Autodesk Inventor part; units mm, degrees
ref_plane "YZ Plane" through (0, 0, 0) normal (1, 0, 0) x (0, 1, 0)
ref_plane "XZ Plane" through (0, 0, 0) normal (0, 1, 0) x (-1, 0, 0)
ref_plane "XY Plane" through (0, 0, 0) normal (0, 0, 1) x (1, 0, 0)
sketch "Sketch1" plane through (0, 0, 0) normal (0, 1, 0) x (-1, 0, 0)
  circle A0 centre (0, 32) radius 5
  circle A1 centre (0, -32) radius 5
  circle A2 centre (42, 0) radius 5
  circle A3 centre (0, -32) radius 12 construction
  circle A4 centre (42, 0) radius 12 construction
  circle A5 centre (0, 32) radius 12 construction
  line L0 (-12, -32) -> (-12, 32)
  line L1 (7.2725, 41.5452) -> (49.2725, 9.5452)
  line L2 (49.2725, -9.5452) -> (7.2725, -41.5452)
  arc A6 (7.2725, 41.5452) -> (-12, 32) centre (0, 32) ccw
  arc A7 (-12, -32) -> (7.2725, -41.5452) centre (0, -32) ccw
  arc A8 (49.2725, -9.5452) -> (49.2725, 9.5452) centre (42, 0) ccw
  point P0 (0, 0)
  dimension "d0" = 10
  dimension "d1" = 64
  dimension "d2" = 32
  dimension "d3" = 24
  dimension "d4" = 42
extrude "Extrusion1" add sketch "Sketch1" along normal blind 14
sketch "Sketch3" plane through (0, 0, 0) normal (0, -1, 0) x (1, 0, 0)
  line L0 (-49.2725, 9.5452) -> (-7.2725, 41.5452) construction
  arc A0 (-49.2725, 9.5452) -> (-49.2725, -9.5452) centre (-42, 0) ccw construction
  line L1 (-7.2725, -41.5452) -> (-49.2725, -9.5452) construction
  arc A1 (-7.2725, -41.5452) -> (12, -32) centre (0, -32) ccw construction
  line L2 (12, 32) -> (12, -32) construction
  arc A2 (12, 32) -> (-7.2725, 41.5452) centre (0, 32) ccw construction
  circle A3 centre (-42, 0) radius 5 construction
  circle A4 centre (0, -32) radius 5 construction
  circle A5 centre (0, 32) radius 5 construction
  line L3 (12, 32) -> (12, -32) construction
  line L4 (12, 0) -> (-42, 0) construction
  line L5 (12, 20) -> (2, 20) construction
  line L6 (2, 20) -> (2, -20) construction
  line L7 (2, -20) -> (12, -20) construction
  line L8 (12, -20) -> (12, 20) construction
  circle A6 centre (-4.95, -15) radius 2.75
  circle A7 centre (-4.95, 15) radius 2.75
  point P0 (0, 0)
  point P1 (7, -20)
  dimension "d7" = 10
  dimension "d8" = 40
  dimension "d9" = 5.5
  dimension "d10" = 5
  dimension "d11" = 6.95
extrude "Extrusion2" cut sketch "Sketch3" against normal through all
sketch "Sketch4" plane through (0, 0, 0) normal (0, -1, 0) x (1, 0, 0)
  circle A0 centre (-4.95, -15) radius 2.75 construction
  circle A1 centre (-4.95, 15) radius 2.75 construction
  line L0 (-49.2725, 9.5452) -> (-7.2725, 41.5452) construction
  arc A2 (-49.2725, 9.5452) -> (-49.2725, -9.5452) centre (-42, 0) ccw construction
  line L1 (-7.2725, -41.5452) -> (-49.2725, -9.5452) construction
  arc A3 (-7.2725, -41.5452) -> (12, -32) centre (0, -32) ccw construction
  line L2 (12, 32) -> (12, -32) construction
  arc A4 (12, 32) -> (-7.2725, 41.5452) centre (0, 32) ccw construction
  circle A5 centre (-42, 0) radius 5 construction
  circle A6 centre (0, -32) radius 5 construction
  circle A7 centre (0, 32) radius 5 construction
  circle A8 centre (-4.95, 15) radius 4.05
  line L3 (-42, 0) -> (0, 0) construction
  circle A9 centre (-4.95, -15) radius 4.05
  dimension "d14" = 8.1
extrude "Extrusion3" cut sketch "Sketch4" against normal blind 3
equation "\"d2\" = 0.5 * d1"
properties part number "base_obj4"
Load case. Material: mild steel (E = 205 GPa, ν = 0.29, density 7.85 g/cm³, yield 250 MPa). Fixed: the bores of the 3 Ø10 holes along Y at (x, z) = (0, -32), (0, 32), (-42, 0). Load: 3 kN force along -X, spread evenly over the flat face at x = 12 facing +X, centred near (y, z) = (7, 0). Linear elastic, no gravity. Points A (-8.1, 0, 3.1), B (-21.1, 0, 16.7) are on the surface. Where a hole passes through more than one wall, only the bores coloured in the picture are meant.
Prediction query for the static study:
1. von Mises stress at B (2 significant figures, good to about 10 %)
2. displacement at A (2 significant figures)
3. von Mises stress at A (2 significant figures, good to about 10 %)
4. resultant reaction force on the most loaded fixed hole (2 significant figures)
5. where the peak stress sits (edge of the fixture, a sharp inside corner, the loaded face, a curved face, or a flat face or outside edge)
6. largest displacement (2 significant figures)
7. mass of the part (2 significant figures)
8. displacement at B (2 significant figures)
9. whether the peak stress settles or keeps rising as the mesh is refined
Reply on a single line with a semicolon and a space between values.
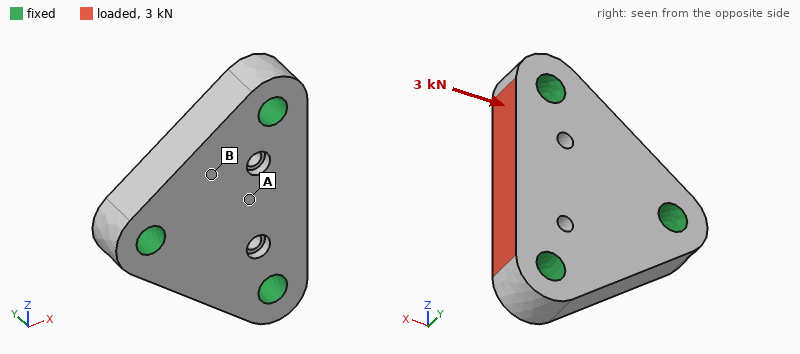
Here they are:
1.2 MPa; 0.46 µm; 3.0 MPa; 1.1 kN; edge of the fixture; 0.76 µm; 390 g; 0.25 µm; keeps rising
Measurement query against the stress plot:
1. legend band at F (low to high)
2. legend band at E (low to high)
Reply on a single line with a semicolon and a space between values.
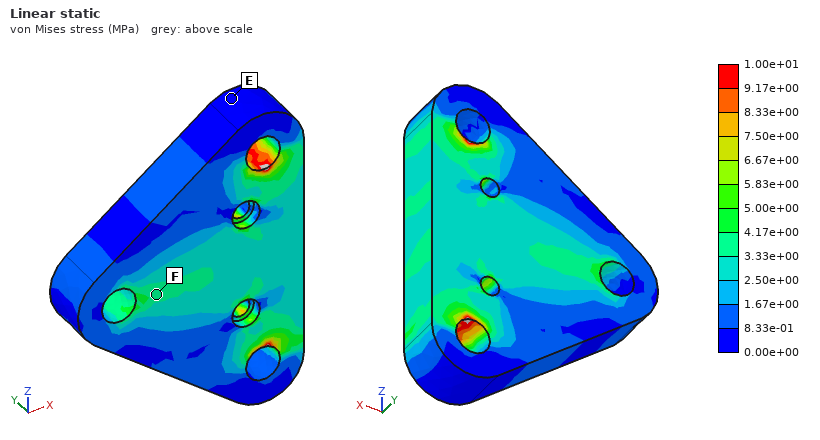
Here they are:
3.33e+00 to 4.17e+00 MPa; 0.00e+00 to 8.33e-01 MPa
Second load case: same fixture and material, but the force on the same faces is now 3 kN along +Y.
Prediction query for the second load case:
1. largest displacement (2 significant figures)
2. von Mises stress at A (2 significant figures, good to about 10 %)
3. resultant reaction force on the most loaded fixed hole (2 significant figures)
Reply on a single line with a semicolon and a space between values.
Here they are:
5.0 µm; 8.9 MPa; 1.6 kN
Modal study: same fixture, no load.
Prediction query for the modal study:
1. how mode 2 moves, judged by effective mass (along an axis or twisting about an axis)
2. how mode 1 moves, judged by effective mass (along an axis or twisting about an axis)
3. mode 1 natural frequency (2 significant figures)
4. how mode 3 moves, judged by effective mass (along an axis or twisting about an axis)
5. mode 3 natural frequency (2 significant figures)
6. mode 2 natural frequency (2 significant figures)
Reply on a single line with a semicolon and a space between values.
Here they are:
along Y; along Y; 16 kHz; twisting about X; 24 kHz; 22 kHz
